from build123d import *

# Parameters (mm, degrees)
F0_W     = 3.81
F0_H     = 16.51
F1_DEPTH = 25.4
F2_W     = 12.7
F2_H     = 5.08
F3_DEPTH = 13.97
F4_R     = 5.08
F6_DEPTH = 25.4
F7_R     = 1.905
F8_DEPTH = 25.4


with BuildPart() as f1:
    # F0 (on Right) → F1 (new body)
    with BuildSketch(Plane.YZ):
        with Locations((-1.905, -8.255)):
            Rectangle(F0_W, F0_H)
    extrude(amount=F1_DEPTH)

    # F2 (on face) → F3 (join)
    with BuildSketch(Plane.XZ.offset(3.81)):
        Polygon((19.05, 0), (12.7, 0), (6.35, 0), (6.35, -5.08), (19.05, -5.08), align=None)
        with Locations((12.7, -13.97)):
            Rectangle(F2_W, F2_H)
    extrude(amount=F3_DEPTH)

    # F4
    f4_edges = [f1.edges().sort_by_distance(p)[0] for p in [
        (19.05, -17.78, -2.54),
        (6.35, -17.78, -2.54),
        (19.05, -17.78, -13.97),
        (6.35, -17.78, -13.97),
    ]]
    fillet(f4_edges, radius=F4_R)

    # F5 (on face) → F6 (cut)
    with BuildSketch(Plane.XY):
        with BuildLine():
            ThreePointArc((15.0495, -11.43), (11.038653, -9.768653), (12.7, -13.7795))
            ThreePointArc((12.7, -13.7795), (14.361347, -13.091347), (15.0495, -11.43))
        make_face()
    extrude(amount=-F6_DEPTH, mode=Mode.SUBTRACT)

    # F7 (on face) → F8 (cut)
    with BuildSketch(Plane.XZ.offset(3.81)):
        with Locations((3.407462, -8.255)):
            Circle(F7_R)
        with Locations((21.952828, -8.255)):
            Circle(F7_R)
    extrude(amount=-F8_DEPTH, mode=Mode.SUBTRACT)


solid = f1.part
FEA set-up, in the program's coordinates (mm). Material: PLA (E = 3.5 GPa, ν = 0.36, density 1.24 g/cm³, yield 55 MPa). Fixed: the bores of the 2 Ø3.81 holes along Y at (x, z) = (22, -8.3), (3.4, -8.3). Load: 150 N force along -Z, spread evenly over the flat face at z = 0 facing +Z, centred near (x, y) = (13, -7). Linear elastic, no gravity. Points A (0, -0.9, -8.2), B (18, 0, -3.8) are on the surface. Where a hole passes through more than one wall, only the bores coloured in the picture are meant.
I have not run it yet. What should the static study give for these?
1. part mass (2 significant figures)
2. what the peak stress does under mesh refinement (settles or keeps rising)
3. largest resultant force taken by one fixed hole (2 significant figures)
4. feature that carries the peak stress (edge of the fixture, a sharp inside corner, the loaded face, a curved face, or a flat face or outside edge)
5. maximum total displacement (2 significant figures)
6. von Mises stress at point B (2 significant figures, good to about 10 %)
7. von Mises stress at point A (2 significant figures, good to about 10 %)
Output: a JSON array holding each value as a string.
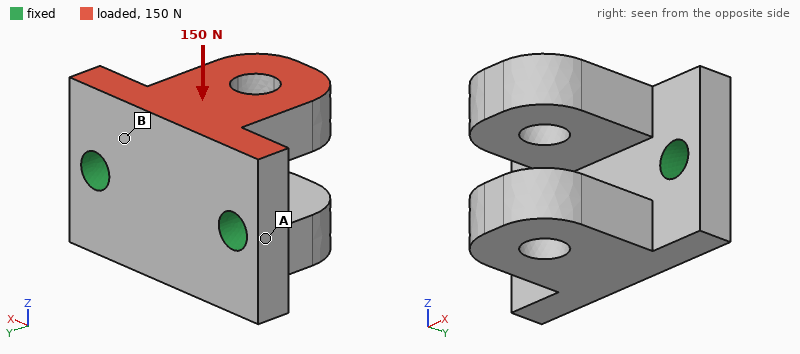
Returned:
["3.8 g", "keeps rising", "77 N", "edge of the fixture", "0.28 mm", "7.7 MPa", "3.3 MPa"]
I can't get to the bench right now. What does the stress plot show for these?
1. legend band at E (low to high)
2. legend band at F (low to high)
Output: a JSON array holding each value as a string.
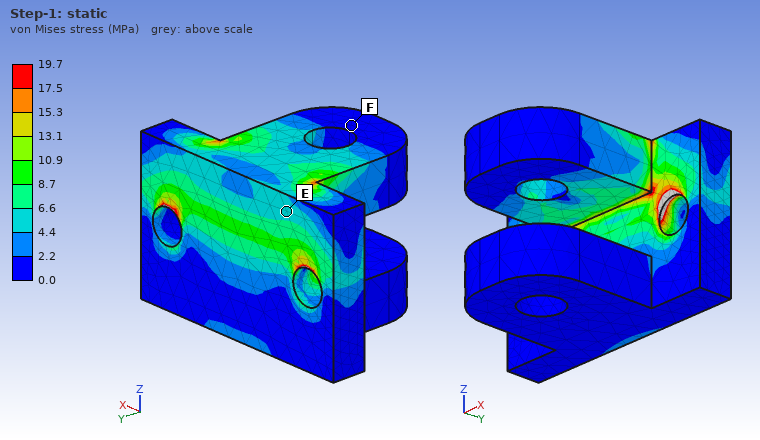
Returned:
["4.4 to 6.6 MPa", "0.0 to 2.2 MPa"]
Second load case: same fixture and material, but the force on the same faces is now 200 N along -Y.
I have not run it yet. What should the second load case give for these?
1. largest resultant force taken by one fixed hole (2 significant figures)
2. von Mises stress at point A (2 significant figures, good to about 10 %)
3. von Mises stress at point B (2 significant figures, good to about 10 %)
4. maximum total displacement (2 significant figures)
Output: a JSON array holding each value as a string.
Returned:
["100 N", "7.2 MPa", "10 MPa", "0.33 mm"]
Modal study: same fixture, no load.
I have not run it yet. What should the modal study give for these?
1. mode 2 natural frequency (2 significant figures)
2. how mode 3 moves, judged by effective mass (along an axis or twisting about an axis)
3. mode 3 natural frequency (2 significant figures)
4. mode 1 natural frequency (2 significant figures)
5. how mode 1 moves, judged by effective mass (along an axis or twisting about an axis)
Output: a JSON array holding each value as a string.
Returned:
["3900 Hz", "along X", "7100 Hz", "3400 Hz", "along Z"]
